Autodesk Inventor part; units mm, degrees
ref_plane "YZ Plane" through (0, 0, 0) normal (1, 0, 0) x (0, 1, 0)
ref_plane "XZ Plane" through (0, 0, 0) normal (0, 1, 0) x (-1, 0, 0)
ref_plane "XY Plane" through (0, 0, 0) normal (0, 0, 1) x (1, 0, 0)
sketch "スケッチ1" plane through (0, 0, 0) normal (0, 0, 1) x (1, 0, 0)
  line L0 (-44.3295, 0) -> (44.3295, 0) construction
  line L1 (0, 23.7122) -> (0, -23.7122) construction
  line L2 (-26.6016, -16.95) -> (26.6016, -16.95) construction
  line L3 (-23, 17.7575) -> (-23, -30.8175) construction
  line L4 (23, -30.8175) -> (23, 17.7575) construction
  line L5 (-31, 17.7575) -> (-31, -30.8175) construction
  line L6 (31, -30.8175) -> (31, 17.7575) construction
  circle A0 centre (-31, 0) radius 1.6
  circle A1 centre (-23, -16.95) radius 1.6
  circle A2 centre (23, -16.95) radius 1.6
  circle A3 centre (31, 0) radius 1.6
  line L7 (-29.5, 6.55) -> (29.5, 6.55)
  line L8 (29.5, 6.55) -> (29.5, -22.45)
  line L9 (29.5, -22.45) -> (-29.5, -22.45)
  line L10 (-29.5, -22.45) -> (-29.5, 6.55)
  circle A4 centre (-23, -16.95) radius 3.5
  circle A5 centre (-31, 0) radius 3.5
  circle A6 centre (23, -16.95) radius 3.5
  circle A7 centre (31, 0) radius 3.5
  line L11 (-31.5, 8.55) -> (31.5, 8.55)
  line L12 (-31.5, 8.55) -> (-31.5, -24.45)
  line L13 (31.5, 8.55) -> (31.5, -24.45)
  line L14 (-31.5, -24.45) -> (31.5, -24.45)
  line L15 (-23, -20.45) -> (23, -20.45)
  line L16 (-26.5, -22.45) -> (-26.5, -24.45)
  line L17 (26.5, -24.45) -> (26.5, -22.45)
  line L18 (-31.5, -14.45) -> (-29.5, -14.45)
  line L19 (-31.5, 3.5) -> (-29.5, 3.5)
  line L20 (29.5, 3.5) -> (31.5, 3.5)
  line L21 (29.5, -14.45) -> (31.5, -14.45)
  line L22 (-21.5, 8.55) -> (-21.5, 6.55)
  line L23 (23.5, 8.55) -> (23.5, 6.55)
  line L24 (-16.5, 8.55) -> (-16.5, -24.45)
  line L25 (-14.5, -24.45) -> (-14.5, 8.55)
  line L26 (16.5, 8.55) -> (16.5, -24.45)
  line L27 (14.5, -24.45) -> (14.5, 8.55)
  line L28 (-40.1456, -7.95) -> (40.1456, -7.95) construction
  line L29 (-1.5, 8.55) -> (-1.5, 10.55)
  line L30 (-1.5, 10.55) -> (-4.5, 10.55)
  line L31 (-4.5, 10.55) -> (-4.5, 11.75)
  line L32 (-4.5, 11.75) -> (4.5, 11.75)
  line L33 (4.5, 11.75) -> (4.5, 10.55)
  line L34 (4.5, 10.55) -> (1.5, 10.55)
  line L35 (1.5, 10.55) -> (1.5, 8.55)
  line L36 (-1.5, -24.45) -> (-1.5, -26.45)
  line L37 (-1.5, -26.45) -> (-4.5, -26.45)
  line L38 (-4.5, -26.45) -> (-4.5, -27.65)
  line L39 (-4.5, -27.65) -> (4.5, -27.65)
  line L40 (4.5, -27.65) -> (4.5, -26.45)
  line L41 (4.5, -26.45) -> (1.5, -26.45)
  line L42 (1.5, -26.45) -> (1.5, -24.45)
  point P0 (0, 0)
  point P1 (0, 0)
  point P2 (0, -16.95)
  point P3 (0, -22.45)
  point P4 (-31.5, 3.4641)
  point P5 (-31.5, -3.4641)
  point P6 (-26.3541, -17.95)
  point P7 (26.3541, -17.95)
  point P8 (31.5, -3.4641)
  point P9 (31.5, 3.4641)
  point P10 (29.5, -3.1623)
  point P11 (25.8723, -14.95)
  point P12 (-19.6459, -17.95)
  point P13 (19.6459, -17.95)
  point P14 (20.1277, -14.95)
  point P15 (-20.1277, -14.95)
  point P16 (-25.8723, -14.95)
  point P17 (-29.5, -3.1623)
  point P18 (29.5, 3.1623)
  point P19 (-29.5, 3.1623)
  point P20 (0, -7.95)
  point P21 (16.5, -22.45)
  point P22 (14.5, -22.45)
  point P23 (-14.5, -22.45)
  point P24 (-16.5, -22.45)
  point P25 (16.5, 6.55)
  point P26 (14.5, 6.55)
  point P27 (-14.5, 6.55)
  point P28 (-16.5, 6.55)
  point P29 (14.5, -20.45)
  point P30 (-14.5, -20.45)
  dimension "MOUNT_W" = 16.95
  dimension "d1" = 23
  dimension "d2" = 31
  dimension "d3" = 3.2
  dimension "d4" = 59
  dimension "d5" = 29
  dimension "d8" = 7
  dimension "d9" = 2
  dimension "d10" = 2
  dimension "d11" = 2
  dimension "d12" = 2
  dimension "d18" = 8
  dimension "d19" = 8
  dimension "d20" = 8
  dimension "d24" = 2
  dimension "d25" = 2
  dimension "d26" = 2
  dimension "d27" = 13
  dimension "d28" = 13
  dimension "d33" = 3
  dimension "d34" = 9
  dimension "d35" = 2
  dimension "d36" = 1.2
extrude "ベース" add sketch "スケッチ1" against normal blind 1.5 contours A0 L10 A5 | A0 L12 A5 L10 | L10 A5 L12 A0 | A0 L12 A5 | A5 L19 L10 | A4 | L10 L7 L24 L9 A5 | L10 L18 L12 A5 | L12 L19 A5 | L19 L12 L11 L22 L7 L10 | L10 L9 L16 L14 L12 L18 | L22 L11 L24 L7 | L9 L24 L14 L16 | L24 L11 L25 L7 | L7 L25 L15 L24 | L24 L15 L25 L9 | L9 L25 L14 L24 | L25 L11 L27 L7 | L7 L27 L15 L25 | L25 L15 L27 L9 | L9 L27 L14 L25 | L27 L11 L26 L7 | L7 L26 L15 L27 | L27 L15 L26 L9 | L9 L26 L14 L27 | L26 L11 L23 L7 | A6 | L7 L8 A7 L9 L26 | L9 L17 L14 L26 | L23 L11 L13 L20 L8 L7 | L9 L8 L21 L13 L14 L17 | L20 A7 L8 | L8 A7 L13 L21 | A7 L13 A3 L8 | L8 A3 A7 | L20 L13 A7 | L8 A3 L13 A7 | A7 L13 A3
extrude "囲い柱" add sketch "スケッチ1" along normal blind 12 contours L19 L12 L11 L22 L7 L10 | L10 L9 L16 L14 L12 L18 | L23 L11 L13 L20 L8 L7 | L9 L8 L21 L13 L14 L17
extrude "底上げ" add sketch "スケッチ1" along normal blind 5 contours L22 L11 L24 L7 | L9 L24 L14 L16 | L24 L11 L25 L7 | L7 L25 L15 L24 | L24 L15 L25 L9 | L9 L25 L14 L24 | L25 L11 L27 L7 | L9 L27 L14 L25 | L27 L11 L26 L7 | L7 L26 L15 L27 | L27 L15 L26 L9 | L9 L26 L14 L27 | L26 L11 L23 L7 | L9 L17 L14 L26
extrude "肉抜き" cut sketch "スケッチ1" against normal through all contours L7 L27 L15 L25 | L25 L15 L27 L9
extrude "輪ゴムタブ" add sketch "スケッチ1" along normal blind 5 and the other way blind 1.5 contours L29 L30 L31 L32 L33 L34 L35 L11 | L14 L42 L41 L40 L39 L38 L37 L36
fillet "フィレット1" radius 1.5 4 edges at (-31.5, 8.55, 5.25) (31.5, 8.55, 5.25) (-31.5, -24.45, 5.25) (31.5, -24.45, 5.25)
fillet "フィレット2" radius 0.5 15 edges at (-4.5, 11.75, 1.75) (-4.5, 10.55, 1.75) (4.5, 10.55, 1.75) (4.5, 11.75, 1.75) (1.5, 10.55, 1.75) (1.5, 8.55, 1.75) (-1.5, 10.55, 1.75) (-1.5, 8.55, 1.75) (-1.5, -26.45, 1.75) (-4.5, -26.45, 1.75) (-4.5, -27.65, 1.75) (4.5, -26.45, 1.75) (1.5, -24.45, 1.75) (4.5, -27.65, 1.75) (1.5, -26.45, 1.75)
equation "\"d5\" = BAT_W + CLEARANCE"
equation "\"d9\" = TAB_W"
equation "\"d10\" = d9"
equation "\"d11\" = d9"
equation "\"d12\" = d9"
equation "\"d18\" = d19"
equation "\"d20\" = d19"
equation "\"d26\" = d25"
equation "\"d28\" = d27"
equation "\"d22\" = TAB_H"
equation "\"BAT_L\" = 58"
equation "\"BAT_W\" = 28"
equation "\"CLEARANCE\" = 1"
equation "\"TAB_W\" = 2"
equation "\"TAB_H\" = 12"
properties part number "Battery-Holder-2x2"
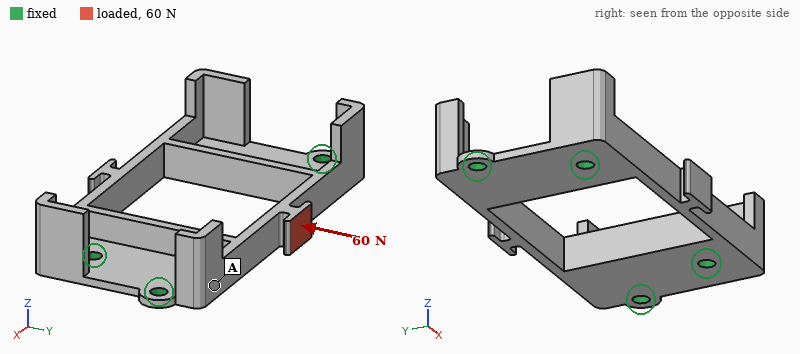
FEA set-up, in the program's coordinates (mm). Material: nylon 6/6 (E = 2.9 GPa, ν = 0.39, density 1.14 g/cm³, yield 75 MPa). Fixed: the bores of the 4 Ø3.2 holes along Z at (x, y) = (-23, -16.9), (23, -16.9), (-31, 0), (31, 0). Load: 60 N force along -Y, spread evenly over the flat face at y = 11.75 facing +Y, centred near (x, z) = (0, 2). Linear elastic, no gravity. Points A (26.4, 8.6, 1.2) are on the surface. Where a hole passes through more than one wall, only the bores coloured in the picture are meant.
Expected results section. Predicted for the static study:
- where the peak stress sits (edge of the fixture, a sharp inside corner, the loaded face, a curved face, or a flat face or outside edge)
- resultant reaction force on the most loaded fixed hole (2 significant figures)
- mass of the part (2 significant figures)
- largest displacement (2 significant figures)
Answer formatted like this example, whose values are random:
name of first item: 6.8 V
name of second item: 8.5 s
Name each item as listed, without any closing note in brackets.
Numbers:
where the peak stress sits: a curved face
resultant reaction force on the most loaded fixed hole: 35 N
mass of the part: 5.5 g
largest displacement: 0.77 mm
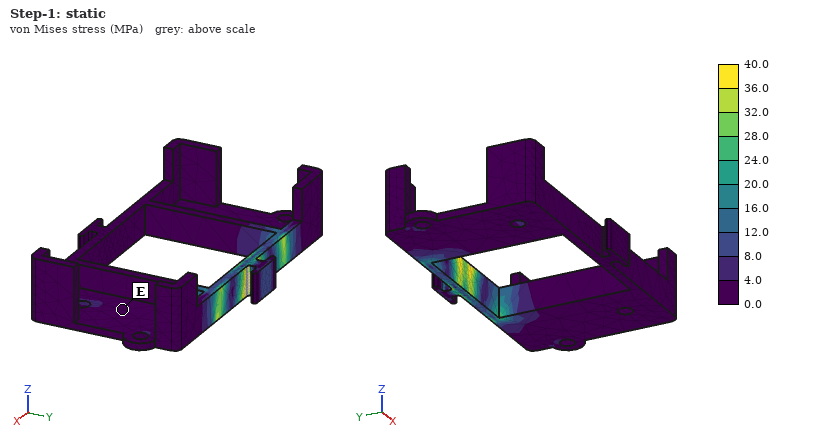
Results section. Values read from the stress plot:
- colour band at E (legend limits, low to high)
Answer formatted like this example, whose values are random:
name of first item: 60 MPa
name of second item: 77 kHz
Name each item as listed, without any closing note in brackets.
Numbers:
colour band at E: 0.0 to 4.0 MPa
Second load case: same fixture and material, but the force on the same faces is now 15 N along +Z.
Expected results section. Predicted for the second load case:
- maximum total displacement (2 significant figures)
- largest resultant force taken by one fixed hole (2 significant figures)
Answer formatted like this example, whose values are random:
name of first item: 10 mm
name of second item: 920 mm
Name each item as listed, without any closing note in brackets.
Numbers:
maximum total displacement: 0.47 mm
largest resultant force taken by one fixed hole: 30 N
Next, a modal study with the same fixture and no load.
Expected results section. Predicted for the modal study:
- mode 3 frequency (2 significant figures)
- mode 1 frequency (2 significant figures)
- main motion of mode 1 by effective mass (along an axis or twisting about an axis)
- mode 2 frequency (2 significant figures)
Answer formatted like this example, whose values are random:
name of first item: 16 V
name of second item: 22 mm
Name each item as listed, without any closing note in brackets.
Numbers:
mode 3 frequency: 2200 Hz
mode 1 frequency: 1200 Hz
main motion of mode 1 by effective mass: along Z
mode 2 frequency: 1900 Hz
